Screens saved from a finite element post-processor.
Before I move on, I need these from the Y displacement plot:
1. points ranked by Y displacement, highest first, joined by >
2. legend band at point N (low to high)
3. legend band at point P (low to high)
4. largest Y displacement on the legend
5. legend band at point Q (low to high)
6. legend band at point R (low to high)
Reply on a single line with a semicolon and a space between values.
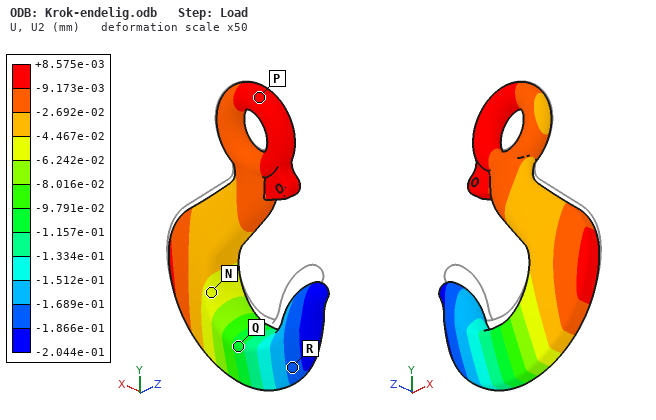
P > N > Q > R; -6.242e-02 to -4.467e-02 mm; -9.173e-03 to +8.575e-03 mm; +8.575e-03 mm; -1.157e-01 to -9.791e-02 mm; -1.866e-01 to -1.689e-01 mm
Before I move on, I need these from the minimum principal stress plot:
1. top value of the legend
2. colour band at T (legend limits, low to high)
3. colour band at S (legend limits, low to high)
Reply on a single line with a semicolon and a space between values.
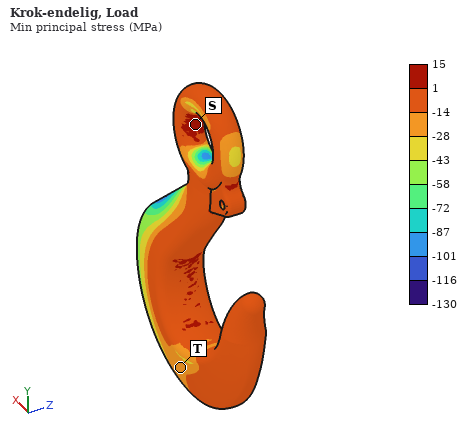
15 MPa; -28 to -14 MPa; 1 to 15 MPa
